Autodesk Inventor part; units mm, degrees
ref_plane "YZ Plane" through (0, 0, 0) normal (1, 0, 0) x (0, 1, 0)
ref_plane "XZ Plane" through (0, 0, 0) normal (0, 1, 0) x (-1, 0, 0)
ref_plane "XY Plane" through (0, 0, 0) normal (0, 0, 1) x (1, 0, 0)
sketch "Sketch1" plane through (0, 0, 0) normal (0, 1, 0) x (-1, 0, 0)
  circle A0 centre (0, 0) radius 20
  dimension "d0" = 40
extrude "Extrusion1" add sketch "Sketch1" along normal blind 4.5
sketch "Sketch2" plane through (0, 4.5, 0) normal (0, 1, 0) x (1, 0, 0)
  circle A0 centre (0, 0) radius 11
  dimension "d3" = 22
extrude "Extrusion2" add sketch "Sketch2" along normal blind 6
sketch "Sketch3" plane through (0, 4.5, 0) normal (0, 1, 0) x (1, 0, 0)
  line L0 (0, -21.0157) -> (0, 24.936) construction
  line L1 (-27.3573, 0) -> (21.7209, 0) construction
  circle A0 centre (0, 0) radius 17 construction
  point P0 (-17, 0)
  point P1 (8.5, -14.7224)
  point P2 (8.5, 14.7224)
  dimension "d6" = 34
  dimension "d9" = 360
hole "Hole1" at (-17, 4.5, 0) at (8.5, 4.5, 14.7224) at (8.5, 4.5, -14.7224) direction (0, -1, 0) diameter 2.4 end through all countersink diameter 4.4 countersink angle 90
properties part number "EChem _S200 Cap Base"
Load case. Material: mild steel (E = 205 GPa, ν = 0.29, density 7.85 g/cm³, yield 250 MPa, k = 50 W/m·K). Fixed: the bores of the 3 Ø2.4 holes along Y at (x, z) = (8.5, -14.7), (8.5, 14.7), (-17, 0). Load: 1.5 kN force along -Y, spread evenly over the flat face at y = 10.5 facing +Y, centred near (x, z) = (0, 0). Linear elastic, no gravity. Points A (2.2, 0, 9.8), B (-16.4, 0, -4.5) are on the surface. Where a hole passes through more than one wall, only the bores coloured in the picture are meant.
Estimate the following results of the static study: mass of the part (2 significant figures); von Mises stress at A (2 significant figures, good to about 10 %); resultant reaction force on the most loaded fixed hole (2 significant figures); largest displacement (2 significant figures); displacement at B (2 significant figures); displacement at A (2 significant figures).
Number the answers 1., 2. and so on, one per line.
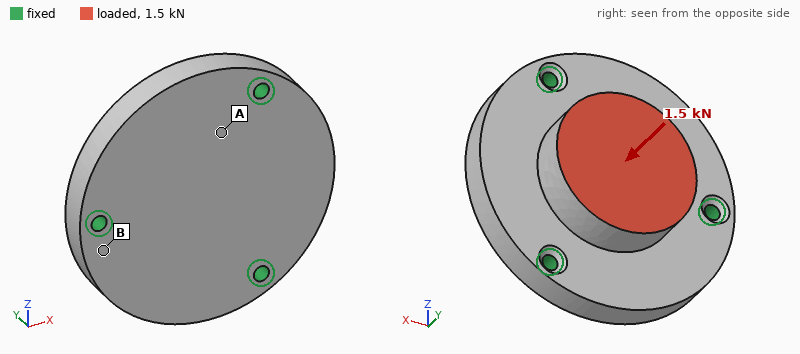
1. 62 g
2. 16 MPa
3. 550 N
4. 3.0 µm
5. 0.95 µm
6. 2.5 µm
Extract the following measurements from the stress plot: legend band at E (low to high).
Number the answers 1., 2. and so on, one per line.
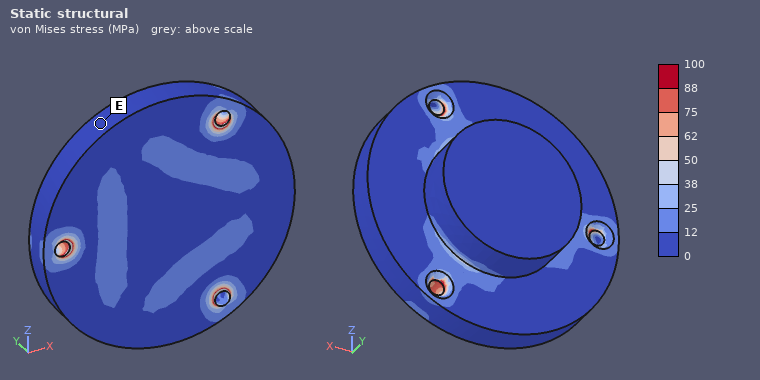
1. 0 to 12 MPa
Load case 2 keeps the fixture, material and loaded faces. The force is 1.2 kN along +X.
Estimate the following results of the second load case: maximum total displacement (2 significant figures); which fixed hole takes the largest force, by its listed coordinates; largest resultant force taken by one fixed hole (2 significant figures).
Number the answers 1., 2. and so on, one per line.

1. 3.2 µm
2. (-17, 0)
3. 670 N
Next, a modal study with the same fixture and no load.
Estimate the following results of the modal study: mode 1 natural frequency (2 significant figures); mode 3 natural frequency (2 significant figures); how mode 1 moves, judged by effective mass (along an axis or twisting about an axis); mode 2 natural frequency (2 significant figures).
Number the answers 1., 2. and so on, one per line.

1. 16 kHz
2. 18 kHz
3. along Y
4. 18 kHz
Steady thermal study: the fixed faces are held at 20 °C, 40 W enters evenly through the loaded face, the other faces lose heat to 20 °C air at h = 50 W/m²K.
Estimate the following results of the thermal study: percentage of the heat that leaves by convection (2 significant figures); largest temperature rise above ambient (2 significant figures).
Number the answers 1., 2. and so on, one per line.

1. 9.6 %
2. 51 K
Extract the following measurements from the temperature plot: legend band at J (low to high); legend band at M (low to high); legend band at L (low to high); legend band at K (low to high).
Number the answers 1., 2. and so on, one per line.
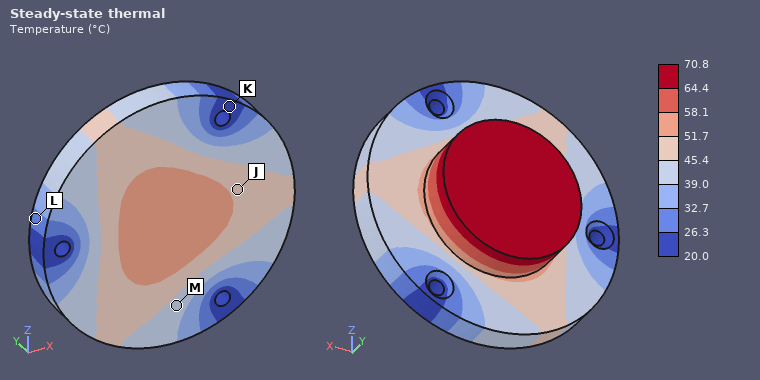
1. 45.4 to 51.7 °C
2. 39.0 to 45.4 °C
3. 26.3 to 32.7 °C
4. 20.0 to 26.3 °C
